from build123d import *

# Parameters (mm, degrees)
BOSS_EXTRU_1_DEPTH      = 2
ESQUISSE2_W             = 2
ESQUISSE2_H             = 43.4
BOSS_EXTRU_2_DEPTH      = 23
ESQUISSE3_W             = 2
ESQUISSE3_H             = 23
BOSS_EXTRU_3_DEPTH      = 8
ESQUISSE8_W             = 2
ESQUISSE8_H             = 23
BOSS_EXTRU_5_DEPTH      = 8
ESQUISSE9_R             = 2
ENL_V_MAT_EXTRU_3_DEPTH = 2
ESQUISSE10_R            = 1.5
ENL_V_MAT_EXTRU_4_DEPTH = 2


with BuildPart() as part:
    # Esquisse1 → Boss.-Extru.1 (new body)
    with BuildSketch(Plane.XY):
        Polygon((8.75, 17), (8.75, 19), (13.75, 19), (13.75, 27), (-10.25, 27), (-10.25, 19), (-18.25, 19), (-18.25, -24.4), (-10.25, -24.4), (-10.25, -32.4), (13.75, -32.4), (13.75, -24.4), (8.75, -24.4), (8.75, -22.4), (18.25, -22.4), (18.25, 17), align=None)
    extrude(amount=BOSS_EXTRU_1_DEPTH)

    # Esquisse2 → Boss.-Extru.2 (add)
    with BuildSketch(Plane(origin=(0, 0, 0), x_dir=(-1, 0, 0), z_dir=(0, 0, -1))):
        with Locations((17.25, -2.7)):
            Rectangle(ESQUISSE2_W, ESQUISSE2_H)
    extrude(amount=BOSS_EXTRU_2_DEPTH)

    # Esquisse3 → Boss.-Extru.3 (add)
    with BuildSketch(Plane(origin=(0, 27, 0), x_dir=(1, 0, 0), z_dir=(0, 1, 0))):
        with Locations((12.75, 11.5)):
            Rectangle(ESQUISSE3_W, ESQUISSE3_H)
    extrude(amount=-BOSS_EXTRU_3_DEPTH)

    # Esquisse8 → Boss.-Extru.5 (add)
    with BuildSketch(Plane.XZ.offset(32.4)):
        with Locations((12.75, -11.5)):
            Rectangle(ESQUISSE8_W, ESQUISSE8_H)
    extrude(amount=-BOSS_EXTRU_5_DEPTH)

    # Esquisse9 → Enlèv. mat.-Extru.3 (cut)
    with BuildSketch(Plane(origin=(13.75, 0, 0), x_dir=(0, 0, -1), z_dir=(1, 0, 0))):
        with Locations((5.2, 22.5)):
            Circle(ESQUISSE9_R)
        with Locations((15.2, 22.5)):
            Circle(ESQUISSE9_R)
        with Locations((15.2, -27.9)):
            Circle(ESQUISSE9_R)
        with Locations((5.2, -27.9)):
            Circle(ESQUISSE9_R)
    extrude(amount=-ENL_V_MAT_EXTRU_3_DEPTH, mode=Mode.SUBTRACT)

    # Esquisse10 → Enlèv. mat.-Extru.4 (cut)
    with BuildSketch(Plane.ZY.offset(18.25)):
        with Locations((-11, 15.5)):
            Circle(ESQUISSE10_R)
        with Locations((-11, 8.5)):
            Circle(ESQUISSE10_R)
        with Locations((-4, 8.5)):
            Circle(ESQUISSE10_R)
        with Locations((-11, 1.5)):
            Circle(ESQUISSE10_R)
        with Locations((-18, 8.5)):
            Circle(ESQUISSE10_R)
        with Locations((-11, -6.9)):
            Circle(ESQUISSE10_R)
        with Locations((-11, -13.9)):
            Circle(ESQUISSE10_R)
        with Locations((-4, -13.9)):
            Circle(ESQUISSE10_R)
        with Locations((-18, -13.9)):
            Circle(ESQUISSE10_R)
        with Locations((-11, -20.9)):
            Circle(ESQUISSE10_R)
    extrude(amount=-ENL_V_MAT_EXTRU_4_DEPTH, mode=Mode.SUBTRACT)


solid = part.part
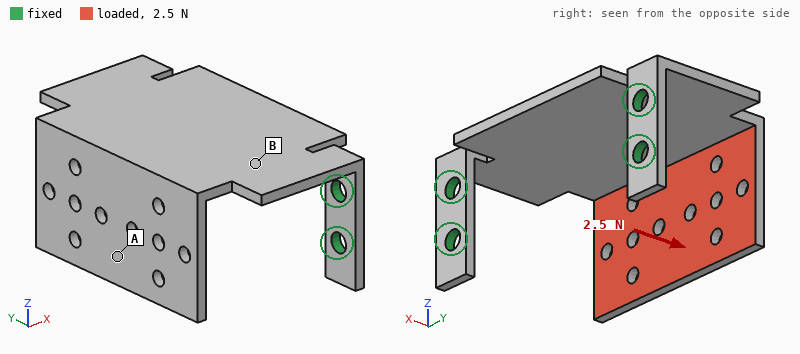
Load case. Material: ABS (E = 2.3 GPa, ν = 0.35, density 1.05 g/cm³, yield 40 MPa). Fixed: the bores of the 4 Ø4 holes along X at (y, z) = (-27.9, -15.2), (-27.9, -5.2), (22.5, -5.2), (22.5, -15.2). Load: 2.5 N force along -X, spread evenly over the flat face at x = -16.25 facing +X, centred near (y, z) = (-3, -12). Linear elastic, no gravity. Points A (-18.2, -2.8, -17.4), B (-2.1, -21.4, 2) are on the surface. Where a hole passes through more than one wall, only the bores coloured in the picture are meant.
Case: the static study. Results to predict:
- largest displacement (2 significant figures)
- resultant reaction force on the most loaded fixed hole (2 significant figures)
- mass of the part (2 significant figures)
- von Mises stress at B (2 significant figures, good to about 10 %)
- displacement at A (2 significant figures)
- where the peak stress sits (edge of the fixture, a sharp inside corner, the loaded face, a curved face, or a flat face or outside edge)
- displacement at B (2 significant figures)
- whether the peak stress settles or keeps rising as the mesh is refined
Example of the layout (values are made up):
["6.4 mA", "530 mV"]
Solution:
["0.78 mm", "1.3 N", "6.7 g", "0.86 MPa", "0.67 mm", "a sharp inside corner", "0.17 mm", "keeps rising"]
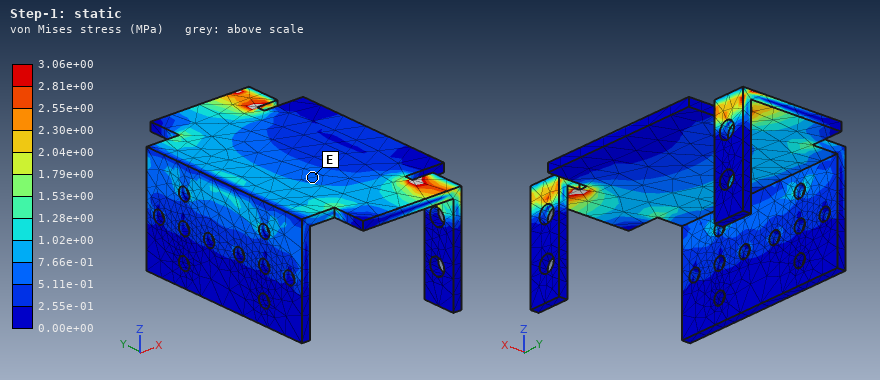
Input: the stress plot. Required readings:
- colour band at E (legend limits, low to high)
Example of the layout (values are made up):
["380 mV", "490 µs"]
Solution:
["5.11e-01 to 7.66e-01 MPa"]
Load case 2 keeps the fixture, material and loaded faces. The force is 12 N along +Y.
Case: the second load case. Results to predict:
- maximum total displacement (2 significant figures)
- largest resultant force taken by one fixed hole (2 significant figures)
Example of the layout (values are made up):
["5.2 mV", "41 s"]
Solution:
["0.87 mm", "9.8 N"]
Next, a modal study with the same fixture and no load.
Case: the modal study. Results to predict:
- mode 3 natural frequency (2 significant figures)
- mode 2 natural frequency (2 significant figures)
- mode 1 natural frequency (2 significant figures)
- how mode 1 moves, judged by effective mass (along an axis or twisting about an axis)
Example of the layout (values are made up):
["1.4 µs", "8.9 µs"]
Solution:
["520 Hz", "410 Hz", "130 Hz", "along Z"]
